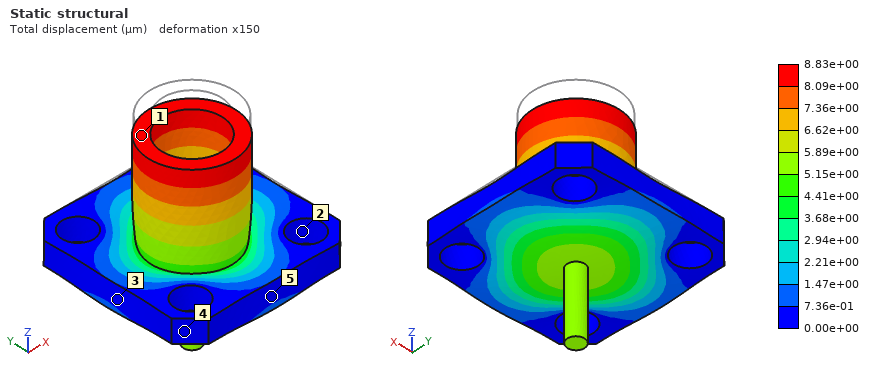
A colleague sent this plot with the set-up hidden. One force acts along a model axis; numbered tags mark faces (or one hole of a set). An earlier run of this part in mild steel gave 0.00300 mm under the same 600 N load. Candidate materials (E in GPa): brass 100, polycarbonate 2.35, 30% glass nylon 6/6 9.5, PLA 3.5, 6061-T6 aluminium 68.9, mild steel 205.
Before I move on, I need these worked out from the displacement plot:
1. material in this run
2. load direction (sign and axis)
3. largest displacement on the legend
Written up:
6061-T6 aluminium
-Z
8.83e+00 µm
